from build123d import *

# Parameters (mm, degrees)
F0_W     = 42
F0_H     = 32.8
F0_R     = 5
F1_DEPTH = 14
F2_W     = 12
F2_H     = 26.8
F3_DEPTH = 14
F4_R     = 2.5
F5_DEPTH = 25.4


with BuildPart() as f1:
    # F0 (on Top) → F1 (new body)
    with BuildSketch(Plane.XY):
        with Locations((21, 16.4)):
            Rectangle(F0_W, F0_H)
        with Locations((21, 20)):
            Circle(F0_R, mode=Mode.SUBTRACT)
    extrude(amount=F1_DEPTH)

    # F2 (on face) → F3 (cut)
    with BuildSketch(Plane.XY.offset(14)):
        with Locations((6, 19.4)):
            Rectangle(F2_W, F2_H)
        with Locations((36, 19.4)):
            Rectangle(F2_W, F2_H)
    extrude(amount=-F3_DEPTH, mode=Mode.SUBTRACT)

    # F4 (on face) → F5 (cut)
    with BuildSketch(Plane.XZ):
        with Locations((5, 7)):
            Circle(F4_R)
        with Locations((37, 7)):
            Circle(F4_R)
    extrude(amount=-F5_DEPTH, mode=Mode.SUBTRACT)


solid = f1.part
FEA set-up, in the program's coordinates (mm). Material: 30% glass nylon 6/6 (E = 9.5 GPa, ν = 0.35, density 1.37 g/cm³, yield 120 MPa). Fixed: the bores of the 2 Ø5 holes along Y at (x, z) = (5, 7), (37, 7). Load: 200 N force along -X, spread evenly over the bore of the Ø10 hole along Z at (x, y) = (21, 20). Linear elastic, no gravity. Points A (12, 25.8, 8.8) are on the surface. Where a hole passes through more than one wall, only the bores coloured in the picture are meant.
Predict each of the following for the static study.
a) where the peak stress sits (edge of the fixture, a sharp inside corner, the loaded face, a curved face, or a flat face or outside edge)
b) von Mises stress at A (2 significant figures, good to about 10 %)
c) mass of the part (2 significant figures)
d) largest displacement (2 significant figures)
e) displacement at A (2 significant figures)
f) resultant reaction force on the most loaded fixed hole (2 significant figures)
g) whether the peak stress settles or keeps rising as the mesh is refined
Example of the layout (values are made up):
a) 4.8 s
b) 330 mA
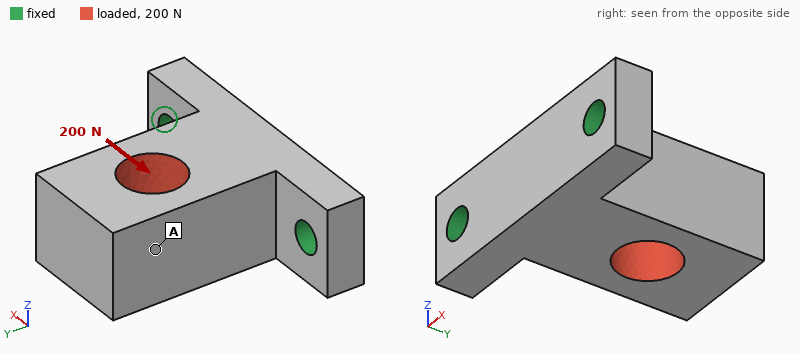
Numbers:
a) edge of the fixture
b) 1.4 MPa
c) 12 g
d) 37 µm
e) 30 µm
f) 170 N
g) keeps rising
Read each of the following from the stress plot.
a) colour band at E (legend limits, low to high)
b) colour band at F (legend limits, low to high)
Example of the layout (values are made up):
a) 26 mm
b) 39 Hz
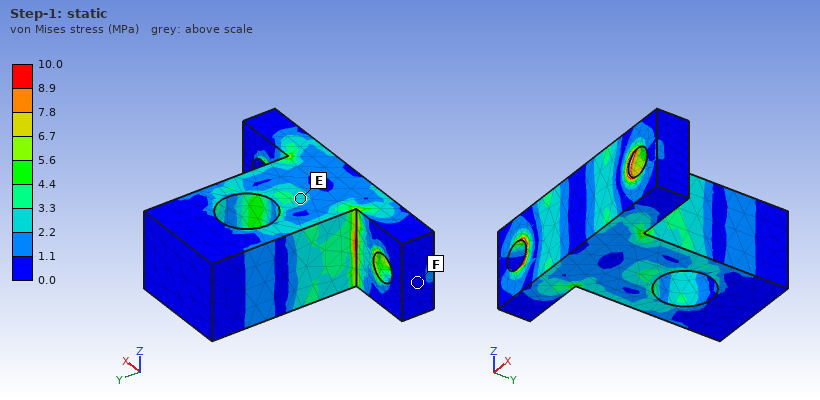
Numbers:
a) 2.2 to 3.3 MPa
b) 0.0 to 1.1 MPa
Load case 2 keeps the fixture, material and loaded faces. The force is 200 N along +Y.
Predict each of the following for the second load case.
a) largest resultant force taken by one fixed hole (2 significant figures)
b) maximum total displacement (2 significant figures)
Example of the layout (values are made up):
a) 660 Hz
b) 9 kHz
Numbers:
a) 110 N
b) 8.0 µm
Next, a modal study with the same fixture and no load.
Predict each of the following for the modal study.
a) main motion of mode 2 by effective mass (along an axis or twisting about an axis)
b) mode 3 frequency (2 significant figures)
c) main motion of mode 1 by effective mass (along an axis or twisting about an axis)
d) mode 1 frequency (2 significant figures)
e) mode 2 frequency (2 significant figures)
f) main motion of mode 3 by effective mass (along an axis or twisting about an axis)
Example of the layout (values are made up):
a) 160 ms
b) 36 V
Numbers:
a) along X
b) 8900 Hz
c) along Z
d) 2500 Hz
e) 4900 Hz
f) along Y
